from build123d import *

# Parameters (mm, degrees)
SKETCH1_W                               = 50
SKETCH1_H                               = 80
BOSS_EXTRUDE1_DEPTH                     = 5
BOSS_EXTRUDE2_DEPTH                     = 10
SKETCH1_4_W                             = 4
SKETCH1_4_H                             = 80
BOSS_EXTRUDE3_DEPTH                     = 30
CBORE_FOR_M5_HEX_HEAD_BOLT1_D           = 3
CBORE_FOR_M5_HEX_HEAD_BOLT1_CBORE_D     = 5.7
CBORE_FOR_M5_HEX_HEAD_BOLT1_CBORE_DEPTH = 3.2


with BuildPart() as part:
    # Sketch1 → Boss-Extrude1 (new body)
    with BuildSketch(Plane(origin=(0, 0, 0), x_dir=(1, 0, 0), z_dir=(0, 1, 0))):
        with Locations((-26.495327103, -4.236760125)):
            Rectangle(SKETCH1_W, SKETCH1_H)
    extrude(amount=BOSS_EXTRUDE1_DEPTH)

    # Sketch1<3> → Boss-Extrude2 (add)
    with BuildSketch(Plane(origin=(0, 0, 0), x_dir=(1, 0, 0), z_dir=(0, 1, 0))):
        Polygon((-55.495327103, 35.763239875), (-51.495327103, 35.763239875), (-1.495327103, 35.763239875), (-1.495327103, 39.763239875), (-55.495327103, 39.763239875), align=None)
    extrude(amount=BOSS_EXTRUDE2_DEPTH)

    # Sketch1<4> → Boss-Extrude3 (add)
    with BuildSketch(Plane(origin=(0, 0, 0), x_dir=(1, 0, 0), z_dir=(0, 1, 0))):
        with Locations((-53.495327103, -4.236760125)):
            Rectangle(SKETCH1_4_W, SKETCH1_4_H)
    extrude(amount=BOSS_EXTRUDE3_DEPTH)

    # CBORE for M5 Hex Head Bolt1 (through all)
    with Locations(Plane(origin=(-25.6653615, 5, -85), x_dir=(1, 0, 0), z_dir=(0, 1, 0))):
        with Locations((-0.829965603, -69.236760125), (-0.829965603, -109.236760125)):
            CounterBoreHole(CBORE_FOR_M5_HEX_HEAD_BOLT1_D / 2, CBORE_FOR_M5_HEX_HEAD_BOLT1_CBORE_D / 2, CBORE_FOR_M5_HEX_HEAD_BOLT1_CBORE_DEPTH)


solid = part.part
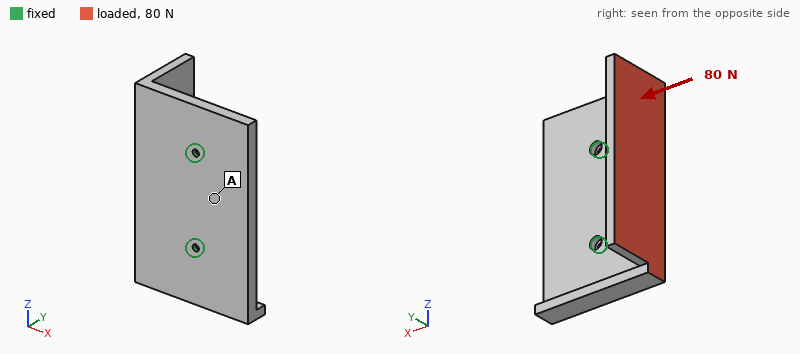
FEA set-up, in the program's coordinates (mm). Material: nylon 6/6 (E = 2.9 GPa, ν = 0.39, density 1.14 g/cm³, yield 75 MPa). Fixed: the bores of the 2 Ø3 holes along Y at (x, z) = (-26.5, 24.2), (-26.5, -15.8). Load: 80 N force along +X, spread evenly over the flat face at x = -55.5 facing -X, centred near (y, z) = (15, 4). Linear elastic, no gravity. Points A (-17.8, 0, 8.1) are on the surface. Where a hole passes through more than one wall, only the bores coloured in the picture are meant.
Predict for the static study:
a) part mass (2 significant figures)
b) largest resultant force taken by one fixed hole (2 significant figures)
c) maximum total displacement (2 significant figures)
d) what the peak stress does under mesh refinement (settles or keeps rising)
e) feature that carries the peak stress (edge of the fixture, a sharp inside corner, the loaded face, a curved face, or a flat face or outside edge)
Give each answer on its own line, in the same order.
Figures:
36 g
41 N
1.2 mm
keeps rising
edge of the fixture
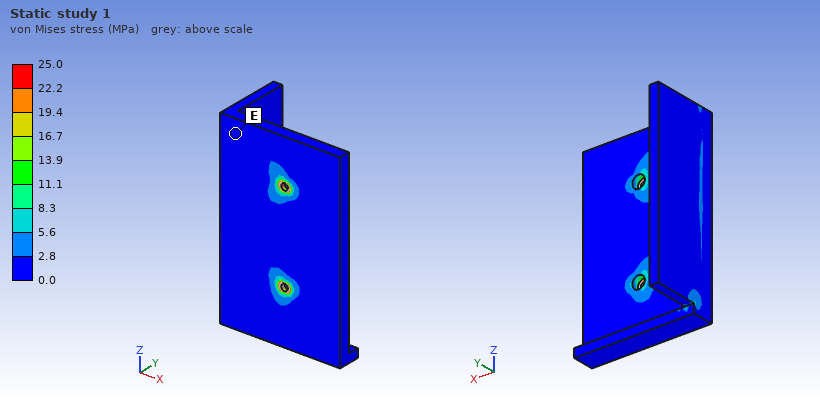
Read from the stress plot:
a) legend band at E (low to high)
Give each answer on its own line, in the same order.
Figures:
0.0 to 2.8 MPa
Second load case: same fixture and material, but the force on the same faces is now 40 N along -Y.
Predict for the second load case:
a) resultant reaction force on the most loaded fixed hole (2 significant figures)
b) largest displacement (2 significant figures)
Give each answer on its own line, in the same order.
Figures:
21 N
1.1 mm
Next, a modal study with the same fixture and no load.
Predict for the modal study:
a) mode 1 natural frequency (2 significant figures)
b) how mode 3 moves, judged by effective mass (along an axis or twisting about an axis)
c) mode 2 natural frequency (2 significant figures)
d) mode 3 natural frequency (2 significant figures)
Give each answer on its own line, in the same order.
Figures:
270 Hz
along Y
670 Hz
1200 Hz
